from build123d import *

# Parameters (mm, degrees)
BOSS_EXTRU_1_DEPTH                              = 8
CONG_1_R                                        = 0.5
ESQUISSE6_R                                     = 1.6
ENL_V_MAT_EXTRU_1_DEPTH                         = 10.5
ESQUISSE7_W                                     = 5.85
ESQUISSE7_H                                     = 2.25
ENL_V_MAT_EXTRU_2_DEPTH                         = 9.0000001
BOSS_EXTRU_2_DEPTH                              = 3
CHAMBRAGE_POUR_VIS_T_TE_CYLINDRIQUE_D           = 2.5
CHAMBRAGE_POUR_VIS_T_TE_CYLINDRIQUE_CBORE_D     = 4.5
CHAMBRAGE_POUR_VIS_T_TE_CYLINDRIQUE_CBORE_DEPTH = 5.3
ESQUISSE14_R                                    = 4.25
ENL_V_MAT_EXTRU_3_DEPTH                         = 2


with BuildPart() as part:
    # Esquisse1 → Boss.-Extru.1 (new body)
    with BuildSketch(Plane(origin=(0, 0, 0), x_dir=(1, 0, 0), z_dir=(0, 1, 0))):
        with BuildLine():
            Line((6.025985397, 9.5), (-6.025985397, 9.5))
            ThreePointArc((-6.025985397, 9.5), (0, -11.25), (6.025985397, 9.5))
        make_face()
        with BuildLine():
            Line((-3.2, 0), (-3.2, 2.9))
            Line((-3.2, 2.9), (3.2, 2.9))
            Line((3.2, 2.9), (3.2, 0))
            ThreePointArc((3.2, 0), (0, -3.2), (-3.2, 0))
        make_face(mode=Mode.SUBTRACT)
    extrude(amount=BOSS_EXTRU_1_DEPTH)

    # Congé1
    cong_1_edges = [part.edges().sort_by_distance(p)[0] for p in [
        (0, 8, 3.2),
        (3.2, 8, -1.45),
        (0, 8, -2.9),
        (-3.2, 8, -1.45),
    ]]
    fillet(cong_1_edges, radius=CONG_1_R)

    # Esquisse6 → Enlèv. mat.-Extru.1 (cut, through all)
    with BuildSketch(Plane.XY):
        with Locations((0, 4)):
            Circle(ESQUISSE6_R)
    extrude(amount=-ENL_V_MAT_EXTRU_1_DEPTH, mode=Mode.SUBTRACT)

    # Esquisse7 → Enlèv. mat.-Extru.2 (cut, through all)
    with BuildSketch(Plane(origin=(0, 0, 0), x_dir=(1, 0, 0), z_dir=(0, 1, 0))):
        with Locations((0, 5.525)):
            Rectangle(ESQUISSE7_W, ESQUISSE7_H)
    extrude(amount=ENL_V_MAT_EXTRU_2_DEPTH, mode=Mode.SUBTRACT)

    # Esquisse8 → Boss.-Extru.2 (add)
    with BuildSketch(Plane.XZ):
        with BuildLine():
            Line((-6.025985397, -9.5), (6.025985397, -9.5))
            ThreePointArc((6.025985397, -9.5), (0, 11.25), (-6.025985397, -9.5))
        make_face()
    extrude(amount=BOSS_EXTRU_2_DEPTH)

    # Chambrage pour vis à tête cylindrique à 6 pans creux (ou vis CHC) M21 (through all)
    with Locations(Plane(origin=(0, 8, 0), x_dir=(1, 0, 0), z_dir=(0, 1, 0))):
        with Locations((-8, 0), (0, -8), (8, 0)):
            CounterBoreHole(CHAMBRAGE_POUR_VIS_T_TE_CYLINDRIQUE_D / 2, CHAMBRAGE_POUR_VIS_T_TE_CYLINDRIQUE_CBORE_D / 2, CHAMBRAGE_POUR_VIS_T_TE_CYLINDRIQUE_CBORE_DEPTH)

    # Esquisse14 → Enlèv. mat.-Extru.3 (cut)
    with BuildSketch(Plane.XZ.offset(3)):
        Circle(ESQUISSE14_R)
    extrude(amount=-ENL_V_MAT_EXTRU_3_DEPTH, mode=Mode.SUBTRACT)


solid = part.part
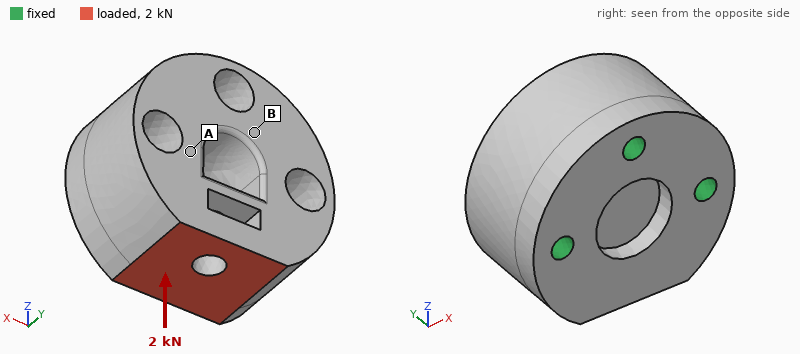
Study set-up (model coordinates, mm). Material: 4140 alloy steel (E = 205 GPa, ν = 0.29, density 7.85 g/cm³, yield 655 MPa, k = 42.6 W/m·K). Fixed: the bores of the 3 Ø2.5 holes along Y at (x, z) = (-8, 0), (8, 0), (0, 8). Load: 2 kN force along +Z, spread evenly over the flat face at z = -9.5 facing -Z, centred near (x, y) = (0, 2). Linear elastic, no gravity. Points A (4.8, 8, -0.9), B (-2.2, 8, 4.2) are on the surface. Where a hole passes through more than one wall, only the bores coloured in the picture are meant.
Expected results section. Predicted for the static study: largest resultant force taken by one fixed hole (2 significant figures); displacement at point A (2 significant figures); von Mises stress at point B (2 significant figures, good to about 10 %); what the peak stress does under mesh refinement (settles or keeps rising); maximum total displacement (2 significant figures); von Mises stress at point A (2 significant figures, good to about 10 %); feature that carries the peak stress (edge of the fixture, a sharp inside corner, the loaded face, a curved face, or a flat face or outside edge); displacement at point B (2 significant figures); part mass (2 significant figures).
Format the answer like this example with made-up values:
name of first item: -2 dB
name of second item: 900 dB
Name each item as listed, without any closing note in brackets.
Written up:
largest resultant force taken by one fixed hole: 860 N
displacement at point A: 1.3 µm
von Mises stress at point B: 9.8 MPa
what the peak stress does under mesh refinement: keeps rising
maximum total displacement: 3.8 µm
von Mises stress at point A: 25 MPa
feature that carries the peak stress: edge of the fixture
displacement at point B: 0.79 µm
part mass: 26 g
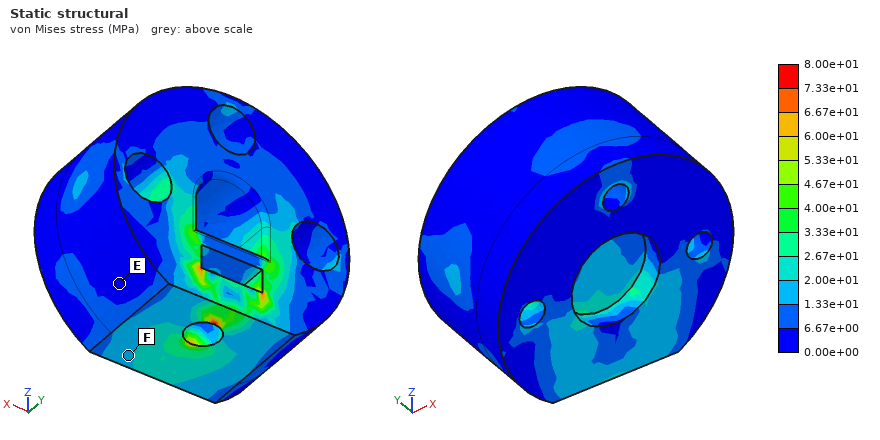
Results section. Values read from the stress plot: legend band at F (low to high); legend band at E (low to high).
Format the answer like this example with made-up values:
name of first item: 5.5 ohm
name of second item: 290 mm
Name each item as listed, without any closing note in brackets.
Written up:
legend band at F: 1.33e+01 to 2.00e+01 MPa
legend band at E: 0.00e+00 to 6.67e+00 MPa
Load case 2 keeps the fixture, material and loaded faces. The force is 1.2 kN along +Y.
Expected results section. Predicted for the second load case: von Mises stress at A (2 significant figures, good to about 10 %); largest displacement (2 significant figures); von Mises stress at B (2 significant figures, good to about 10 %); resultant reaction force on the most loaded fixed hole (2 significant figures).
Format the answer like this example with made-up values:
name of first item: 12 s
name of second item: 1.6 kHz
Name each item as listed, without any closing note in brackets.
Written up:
von Mises stress at A: 42 MPa
largest displacement: 6.7 µm
von Mises stress at B: 17 MPa
resultant reaction force on the most loaded fixed hole: 860 N
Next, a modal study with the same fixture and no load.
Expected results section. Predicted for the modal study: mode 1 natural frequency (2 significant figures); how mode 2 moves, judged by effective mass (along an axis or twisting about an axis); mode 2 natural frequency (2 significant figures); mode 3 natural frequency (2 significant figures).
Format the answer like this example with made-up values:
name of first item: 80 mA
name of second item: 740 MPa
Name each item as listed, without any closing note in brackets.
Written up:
mode 1 natural frequency: 34 kHz
how mode 2 moves, judged by effective mass: along X
mode 2 natural frequency: 50 kHz
mode 3 natural frequency: 56 kHz
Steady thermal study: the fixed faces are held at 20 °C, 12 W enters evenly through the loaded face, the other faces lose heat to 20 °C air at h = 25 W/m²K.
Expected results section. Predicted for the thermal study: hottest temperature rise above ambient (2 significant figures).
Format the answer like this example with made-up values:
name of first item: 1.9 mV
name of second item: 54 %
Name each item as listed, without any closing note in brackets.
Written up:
hottest temperature rise above ambient: 27 K
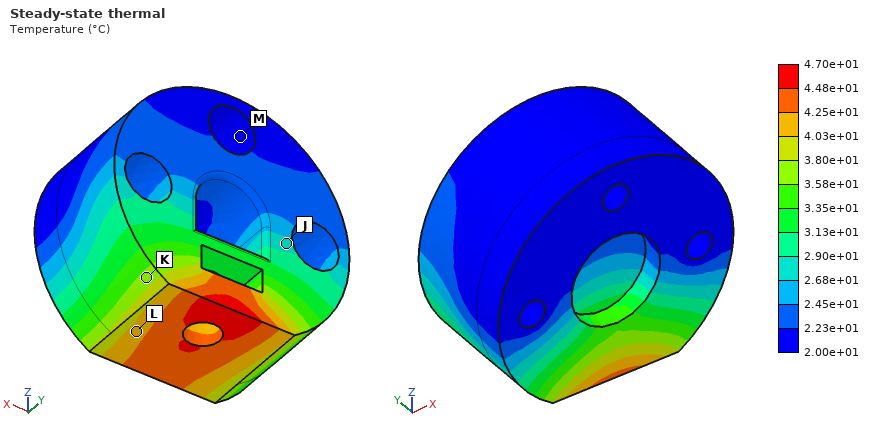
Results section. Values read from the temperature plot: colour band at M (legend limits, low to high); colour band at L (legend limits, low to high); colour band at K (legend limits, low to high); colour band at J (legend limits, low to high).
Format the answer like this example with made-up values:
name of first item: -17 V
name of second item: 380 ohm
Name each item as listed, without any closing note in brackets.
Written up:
colour band at M: 2.00e+01 to 2.23e+01 °C
colour band at L: 4.03e+01 to 4.25e+01 °C
colour band at K: 3.58e+01 to 3.80e+01 °C
colour band at J: 2.68e+01 to 2.90e+01 °C
